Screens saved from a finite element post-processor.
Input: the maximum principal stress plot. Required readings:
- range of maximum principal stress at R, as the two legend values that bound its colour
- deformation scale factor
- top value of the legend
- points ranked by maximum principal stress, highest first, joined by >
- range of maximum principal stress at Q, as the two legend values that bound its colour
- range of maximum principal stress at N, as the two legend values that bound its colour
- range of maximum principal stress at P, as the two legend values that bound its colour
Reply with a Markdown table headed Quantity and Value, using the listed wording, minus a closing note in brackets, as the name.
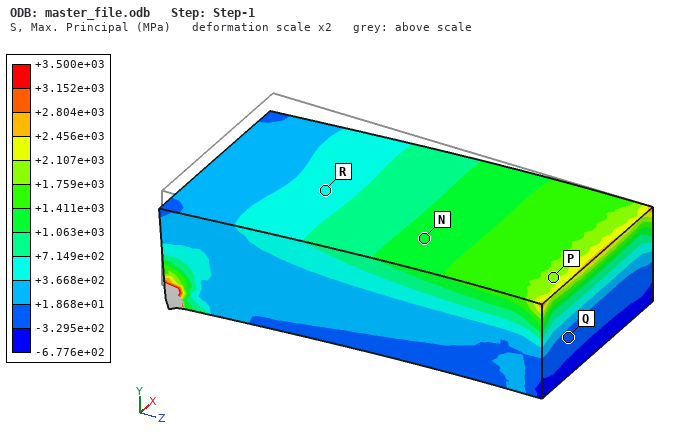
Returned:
| Quantity | Value |
|---|---|
| range of maximum principal stress at R, as the two legend values that bound its colour | +3.668e+02 to +7.149e+02 MPa |
| deformation scale factor | 2 |
| top value of the legend | +3.500e+03 MPa |
| points ranked by maximum principal stress, highest first, joined by > | P > N > R > Q |
| range of maximum principal stress at Q, as the two legend values that bound its colour | -3.295e+02 to +1.868e+01 MPa |
| range of maximum principal stress at N, as the two legend values that bound its colour | +1.063e+03 to +1.411e+03 MPa |
| range of maximum principal stress at P, as the two legend values that bound its colour | +1.759e+03 to +2.107e+03 MPa |
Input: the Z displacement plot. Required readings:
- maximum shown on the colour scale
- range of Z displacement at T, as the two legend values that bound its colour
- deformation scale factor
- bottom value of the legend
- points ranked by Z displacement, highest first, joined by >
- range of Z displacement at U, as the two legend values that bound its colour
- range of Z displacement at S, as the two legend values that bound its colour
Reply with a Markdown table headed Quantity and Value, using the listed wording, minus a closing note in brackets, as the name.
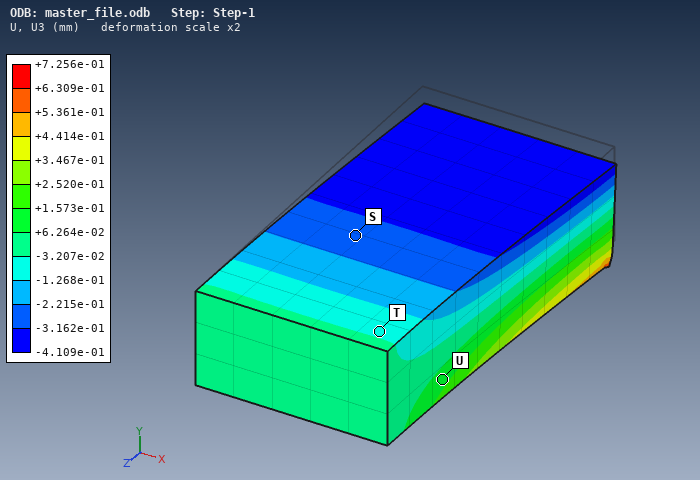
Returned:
| Quantity | Value |
|---|---|
| maximum shown on the colour scale | +7.256e-01 mm |
| range of Z displacement at T, as the two legend values that bound its colour | -1.268e-01 to -3.207e-02 mm |
| deformation scale factor | 2 |
| bottom value of the legend | -4.109e-01 mm |
| points ranked by Z displacement, highest first, joined by > | U > T > S |
| range of Z displacement at U, as the two legend values that bound its colour | +6.264e-02 to +1.573e-01 mm |
| range of Z displacement at S, as the two legend values that bound its colour | -3.162e-01 to -2.215e-01 mm |
